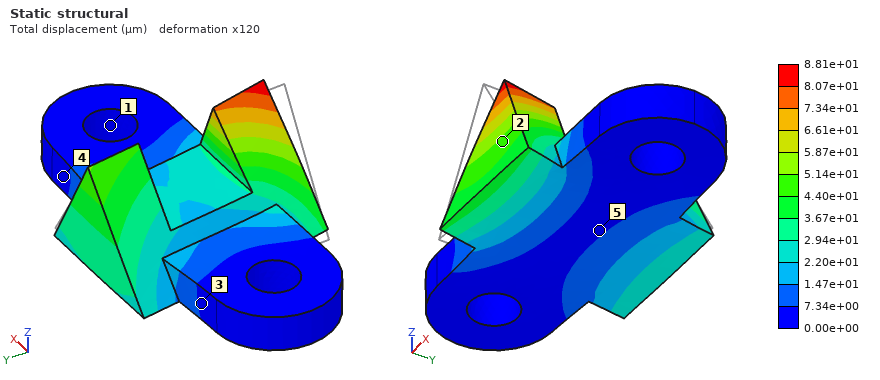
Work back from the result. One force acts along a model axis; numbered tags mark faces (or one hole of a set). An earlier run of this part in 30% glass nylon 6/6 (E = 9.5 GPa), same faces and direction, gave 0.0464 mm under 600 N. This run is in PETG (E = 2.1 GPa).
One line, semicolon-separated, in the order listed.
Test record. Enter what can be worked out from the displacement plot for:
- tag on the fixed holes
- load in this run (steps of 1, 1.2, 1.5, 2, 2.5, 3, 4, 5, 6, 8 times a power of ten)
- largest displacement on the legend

1; 250 N; 8.81e+01 µm
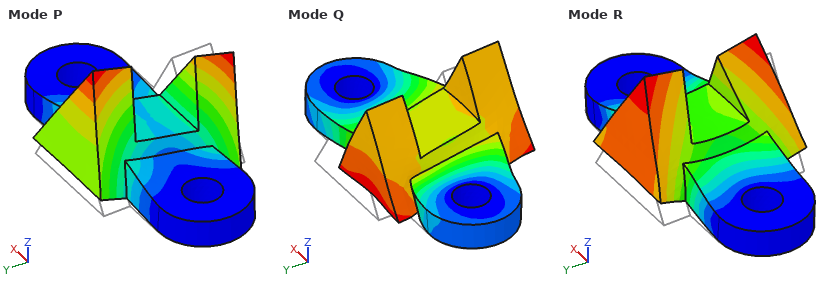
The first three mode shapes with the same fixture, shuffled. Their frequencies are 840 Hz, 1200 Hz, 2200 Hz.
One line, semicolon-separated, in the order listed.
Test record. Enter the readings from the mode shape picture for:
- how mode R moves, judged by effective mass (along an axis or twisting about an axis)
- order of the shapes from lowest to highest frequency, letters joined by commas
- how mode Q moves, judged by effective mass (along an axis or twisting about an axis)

along Z; P, R, Q; along Y
